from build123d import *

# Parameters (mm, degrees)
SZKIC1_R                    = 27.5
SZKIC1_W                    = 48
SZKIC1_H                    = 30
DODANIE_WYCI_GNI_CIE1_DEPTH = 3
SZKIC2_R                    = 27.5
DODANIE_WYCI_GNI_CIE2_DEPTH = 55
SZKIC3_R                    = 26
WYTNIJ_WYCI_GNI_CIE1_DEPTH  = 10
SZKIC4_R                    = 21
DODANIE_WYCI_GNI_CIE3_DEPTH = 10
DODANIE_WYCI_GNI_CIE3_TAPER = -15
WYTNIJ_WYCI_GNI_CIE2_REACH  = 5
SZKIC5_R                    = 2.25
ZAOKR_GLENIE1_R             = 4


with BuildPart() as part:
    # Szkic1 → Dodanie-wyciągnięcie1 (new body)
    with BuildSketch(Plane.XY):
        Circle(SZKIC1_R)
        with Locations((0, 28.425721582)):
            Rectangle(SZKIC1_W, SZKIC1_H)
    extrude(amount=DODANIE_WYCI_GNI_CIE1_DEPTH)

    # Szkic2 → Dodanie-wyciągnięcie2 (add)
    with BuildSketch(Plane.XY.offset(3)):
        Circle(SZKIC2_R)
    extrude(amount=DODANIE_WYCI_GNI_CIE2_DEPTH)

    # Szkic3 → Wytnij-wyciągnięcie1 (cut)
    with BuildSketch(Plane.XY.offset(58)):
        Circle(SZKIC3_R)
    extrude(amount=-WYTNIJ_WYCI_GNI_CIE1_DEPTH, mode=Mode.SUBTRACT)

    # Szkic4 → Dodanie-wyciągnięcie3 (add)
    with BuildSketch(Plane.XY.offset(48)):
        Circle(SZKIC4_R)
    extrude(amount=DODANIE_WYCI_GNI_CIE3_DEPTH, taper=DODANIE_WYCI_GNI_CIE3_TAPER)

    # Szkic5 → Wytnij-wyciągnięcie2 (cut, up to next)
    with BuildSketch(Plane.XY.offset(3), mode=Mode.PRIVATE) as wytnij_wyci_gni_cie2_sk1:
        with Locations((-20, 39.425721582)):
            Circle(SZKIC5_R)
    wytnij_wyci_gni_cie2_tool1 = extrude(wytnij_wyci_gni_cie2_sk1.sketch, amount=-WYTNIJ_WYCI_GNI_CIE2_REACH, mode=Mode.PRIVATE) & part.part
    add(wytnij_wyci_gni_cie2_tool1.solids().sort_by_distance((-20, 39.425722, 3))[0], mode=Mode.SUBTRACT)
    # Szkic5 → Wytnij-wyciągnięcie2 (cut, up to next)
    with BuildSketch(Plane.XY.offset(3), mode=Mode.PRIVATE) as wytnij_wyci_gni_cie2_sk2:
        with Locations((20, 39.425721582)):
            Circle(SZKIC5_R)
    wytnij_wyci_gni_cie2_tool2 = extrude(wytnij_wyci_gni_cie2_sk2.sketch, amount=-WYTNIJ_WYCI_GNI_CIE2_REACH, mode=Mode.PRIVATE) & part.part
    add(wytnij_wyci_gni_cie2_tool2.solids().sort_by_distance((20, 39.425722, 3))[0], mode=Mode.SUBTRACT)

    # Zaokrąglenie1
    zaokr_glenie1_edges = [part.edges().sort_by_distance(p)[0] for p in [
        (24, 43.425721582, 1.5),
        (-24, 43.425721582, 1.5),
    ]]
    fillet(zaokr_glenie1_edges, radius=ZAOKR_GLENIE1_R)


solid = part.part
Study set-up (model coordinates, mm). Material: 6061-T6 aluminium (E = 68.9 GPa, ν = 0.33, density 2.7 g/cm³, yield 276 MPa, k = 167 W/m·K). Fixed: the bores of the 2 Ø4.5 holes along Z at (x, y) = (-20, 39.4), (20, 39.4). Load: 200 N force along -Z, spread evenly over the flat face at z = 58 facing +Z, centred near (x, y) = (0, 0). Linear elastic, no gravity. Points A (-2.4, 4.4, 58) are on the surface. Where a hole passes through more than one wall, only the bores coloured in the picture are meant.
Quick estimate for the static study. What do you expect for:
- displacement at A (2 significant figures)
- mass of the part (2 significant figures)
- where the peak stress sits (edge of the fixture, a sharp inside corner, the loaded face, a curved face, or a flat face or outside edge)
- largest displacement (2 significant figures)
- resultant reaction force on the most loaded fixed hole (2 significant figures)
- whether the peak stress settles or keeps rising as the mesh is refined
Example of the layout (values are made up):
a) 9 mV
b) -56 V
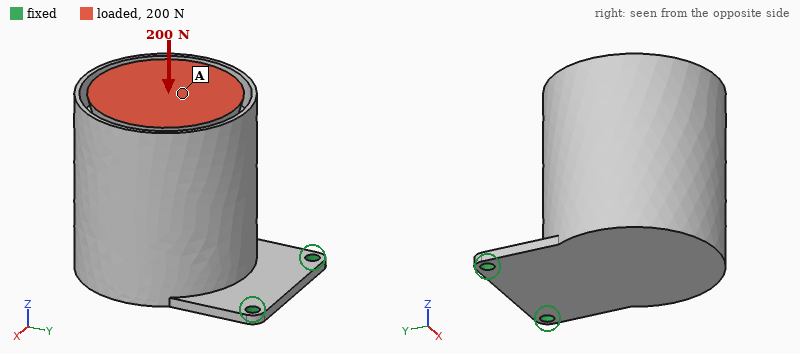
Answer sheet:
a) 0.89 mm
b) 360 g
c) edge of the fixture
d) 1.2 mm
e) 110 N
f) keeps rising
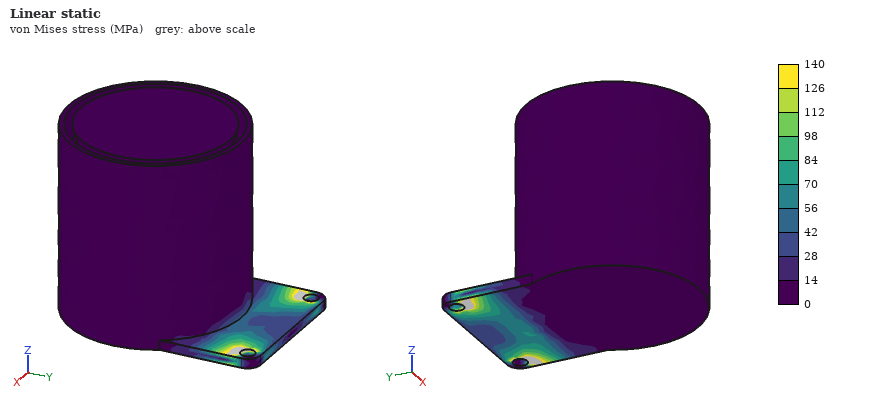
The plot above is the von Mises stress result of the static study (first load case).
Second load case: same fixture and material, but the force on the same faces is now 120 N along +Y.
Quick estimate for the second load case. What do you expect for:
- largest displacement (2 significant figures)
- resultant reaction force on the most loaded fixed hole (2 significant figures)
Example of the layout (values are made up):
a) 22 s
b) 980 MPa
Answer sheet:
a) 1.2 mm
b) 85 N
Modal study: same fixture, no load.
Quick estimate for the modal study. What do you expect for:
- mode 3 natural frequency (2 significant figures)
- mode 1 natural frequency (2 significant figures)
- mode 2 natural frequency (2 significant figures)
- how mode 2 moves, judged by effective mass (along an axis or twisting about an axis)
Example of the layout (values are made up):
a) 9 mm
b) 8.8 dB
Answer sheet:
a) 1300 Hz
b) 120 Hz
c) 470 Hz
d) along X
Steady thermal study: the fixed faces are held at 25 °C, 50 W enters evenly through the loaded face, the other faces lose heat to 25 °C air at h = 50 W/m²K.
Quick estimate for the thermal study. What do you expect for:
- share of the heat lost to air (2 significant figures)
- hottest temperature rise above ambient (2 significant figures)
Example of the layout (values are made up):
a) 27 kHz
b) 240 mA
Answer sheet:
a) 50 %
b) 34 K
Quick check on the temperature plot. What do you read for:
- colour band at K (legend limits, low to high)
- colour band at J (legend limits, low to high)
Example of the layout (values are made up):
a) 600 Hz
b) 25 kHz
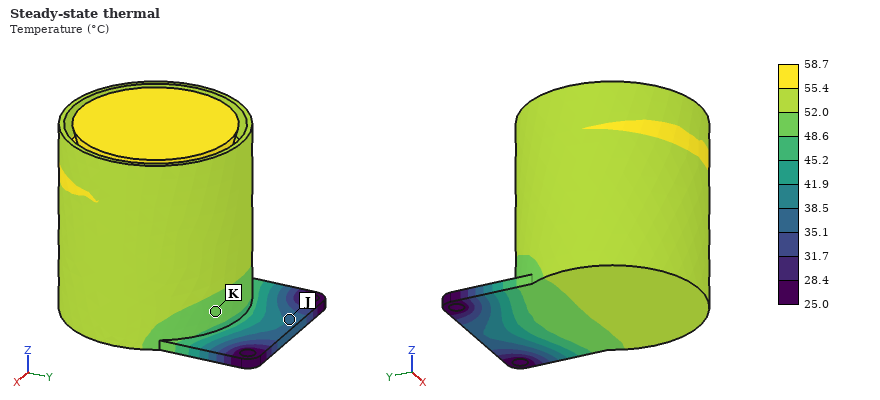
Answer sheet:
a) 48.6 to 52.0 °C
b) 35.1 to 38.5 °C
